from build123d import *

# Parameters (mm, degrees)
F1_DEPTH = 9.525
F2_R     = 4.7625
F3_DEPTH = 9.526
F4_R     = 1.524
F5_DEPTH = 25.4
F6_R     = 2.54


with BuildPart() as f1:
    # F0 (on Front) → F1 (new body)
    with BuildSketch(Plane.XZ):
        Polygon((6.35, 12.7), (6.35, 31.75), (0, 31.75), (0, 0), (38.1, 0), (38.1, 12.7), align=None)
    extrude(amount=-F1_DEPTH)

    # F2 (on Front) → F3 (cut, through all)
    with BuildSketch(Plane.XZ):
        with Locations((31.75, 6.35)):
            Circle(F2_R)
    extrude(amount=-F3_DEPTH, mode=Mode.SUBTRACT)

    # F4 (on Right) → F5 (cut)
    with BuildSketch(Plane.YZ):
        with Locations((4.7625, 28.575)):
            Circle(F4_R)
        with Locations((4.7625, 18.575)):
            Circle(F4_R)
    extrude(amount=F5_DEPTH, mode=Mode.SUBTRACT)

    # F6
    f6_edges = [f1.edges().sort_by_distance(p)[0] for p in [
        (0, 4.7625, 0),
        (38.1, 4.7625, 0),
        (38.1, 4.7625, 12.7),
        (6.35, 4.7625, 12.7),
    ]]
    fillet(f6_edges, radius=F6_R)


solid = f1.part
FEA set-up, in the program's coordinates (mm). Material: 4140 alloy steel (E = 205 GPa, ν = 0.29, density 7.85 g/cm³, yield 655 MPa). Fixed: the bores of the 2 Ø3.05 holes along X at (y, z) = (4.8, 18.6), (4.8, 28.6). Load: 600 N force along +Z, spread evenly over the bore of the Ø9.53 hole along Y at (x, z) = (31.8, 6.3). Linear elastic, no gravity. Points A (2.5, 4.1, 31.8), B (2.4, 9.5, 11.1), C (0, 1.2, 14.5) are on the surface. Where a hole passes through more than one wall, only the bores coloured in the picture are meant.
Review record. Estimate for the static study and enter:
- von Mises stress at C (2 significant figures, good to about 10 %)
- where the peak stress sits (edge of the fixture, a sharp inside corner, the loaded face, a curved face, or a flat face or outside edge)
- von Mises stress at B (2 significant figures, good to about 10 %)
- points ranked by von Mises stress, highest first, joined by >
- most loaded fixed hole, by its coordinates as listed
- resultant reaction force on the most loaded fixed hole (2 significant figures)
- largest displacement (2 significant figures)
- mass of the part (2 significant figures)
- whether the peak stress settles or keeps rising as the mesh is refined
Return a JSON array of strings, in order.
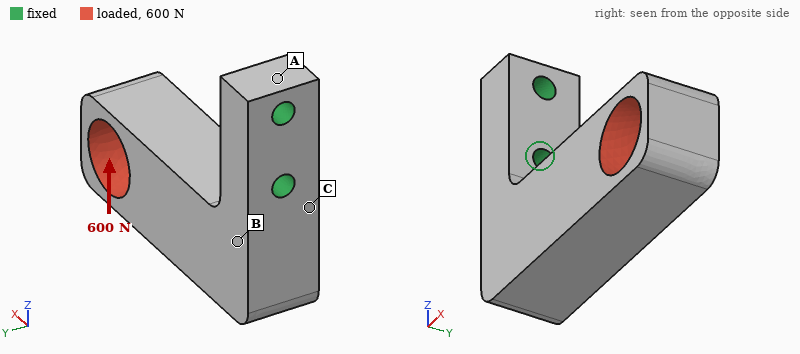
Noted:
["210 MPa", "edge of the fixture", "91 MPa", "C > B > A", "(4.8, 18.6)", "620 N", "0.14 mm", "39 g", "keeps rising"]
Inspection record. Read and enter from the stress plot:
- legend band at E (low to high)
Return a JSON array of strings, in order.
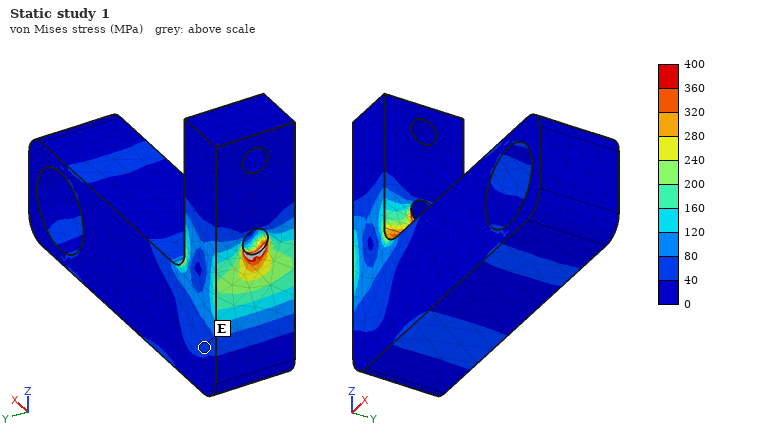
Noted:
["40 to 80 MPa"]
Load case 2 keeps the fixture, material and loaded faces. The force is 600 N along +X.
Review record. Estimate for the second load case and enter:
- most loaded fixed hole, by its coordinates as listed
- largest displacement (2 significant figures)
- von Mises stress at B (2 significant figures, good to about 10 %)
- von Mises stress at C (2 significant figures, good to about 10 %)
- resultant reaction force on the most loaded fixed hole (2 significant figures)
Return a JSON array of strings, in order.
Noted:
["(4.8, 18.6)", "35 µm", "28 MPa", "63 MPa", "710 N"]
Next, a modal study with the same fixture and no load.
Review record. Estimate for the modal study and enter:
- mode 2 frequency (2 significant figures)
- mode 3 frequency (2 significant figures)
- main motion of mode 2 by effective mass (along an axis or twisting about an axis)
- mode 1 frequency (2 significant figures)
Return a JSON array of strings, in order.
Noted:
["3500 Hz", "10 kHz", "along Y", "3400 Hz"]
